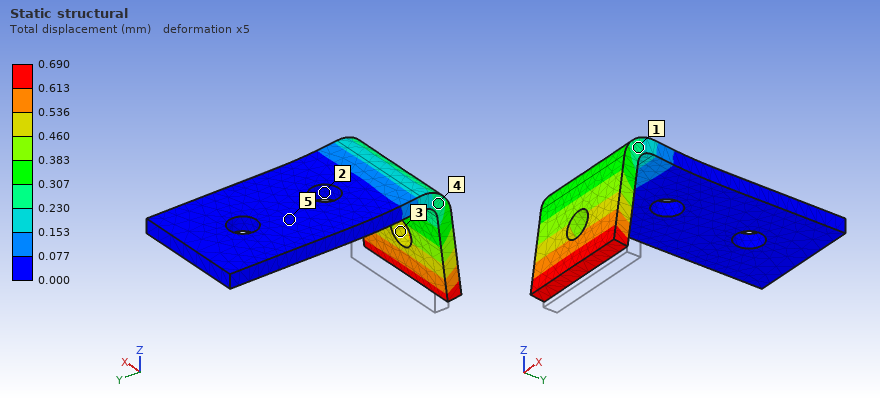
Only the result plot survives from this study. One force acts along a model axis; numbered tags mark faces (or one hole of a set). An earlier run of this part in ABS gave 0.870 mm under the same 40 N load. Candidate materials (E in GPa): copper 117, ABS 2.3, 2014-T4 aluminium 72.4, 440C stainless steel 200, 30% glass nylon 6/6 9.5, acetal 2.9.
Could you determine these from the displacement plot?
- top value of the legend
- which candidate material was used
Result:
0.690 mm
acetal
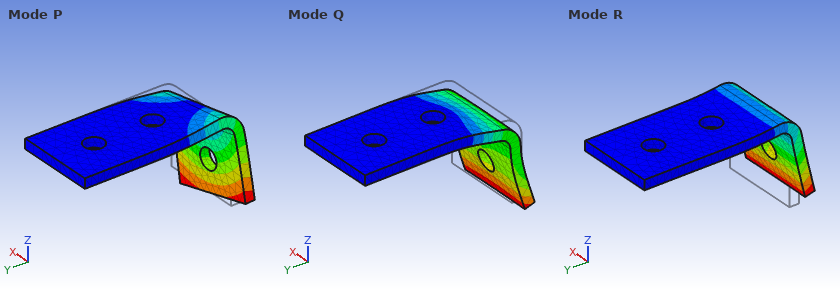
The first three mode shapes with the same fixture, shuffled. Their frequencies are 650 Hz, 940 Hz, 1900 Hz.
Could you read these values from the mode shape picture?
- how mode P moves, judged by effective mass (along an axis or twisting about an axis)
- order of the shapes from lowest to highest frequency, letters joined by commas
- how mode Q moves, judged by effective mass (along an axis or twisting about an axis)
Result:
along X
R, P, Q
along Z
